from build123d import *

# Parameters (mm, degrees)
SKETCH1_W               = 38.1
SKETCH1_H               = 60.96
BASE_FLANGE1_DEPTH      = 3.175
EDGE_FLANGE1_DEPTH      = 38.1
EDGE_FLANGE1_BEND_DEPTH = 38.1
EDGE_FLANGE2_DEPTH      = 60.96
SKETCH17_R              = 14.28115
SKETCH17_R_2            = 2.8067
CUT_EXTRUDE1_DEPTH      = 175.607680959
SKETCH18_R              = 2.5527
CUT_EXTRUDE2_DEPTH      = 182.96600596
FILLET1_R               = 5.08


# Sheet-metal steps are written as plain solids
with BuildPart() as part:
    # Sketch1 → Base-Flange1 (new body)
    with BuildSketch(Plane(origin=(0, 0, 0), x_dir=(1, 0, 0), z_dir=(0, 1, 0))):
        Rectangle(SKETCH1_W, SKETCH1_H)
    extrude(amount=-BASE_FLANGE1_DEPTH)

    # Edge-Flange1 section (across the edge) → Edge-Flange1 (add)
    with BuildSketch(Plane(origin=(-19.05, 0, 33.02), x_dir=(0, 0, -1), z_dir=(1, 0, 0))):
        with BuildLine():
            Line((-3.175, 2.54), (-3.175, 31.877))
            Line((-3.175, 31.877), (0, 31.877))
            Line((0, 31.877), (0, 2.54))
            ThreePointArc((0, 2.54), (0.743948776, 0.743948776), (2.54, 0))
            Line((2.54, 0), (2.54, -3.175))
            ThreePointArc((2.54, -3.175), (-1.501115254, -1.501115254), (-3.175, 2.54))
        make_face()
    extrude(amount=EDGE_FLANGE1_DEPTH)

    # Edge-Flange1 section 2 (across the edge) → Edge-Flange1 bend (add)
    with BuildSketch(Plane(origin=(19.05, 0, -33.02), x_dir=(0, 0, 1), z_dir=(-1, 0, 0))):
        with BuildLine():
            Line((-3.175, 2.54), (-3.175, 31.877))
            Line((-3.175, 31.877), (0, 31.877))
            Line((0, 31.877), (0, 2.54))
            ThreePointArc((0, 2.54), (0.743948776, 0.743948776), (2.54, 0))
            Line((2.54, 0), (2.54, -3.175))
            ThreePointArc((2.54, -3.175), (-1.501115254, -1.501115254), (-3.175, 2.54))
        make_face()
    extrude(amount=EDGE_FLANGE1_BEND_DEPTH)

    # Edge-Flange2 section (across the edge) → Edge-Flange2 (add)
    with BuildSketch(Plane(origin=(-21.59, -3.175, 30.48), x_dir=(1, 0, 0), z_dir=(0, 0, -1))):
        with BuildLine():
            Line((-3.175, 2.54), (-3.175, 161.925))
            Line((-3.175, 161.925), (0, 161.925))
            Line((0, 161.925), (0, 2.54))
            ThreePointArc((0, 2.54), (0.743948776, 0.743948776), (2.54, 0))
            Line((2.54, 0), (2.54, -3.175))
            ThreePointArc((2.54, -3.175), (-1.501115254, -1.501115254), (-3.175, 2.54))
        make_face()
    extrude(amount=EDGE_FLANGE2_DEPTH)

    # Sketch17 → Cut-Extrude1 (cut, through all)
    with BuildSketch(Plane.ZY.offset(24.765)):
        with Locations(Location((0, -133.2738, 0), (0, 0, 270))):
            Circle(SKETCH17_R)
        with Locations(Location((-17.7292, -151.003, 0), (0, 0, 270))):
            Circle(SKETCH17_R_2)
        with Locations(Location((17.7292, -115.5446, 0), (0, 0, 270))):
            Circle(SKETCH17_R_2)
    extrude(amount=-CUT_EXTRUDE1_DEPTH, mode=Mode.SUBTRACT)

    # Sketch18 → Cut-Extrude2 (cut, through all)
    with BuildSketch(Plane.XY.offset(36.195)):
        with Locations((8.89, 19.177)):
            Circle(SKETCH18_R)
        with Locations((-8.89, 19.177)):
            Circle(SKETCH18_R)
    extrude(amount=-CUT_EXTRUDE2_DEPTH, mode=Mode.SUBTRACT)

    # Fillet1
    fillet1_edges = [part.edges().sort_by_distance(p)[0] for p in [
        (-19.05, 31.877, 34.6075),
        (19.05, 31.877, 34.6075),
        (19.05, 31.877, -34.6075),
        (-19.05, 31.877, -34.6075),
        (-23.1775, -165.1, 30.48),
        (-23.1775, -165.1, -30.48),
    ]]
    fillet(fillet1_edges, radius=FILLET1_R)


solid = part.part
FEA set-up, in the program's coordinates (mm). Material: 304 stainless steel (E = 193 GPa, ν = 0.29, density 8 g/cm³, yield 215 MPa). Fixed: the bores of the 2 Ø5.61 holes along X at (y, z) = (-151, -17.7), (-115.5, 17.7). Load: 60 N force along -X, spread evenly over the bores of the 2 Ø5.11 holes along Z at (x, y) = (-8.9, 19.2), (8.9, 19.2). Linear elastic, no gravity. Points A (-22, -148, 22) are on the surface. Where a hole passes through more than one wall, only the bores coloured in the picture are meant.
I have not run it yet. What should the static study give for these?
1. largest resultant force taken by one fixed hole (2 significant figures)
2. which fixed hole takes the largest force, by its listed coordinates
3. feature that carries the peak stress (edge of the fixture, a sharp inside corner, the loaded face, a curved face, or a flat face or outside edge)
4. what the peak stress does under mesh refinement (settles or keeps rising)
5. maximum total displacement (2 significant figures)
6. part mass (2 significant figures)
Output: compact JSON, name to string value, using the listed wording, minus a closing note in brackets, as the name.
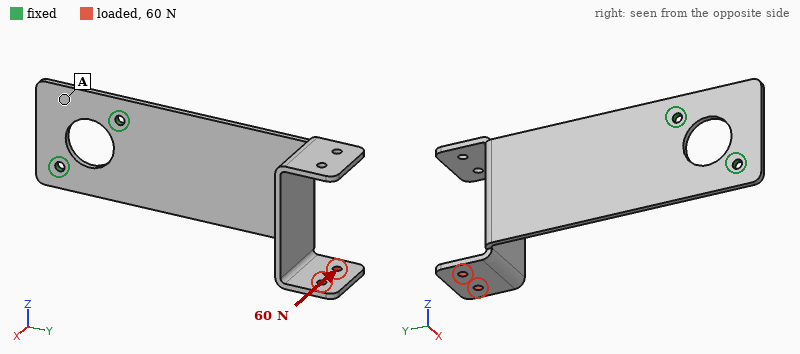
{"largest resultant force taken by one fixed hole": "110 N", "which fixed hole takes the largest force, by its listed coordinates": "(-115.5, 17.7)", "feature that carries the peak stress": "edge of the fixture", "what the peak stress does under mesh refinement": "keeps rising", "maximum total displacement": "2.5 mm", "part mass": "360 g"}
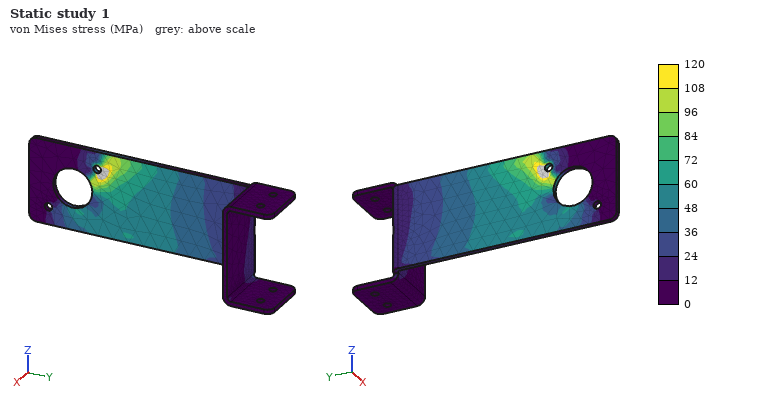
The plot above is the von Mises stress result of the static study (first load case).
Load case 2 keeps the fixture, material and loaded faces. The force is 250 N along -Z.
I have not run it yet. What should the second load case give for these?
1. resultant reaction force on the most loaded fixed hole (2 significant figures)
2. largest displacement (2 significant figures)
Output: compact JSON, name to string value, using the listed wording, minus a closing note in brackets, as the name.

{"resultant reaction force on the most loaded fixed hole": "810 N", "largest displacement": "1.0 mm"}
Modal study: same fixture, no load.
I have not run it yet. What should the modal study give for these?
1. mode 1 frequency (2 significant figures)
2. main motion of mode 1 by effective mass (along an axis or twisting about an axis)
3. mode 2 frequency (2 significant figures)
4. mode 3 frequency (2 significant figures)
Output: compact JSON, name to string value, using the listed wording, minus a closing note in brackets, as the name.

{"mode 1 frequency": "80 Hz", "main motion of mode 1 by effective mass": "along X", "mode 2 frequency": "230 Hz", "mode 3 frequency": "430 Hz"}
